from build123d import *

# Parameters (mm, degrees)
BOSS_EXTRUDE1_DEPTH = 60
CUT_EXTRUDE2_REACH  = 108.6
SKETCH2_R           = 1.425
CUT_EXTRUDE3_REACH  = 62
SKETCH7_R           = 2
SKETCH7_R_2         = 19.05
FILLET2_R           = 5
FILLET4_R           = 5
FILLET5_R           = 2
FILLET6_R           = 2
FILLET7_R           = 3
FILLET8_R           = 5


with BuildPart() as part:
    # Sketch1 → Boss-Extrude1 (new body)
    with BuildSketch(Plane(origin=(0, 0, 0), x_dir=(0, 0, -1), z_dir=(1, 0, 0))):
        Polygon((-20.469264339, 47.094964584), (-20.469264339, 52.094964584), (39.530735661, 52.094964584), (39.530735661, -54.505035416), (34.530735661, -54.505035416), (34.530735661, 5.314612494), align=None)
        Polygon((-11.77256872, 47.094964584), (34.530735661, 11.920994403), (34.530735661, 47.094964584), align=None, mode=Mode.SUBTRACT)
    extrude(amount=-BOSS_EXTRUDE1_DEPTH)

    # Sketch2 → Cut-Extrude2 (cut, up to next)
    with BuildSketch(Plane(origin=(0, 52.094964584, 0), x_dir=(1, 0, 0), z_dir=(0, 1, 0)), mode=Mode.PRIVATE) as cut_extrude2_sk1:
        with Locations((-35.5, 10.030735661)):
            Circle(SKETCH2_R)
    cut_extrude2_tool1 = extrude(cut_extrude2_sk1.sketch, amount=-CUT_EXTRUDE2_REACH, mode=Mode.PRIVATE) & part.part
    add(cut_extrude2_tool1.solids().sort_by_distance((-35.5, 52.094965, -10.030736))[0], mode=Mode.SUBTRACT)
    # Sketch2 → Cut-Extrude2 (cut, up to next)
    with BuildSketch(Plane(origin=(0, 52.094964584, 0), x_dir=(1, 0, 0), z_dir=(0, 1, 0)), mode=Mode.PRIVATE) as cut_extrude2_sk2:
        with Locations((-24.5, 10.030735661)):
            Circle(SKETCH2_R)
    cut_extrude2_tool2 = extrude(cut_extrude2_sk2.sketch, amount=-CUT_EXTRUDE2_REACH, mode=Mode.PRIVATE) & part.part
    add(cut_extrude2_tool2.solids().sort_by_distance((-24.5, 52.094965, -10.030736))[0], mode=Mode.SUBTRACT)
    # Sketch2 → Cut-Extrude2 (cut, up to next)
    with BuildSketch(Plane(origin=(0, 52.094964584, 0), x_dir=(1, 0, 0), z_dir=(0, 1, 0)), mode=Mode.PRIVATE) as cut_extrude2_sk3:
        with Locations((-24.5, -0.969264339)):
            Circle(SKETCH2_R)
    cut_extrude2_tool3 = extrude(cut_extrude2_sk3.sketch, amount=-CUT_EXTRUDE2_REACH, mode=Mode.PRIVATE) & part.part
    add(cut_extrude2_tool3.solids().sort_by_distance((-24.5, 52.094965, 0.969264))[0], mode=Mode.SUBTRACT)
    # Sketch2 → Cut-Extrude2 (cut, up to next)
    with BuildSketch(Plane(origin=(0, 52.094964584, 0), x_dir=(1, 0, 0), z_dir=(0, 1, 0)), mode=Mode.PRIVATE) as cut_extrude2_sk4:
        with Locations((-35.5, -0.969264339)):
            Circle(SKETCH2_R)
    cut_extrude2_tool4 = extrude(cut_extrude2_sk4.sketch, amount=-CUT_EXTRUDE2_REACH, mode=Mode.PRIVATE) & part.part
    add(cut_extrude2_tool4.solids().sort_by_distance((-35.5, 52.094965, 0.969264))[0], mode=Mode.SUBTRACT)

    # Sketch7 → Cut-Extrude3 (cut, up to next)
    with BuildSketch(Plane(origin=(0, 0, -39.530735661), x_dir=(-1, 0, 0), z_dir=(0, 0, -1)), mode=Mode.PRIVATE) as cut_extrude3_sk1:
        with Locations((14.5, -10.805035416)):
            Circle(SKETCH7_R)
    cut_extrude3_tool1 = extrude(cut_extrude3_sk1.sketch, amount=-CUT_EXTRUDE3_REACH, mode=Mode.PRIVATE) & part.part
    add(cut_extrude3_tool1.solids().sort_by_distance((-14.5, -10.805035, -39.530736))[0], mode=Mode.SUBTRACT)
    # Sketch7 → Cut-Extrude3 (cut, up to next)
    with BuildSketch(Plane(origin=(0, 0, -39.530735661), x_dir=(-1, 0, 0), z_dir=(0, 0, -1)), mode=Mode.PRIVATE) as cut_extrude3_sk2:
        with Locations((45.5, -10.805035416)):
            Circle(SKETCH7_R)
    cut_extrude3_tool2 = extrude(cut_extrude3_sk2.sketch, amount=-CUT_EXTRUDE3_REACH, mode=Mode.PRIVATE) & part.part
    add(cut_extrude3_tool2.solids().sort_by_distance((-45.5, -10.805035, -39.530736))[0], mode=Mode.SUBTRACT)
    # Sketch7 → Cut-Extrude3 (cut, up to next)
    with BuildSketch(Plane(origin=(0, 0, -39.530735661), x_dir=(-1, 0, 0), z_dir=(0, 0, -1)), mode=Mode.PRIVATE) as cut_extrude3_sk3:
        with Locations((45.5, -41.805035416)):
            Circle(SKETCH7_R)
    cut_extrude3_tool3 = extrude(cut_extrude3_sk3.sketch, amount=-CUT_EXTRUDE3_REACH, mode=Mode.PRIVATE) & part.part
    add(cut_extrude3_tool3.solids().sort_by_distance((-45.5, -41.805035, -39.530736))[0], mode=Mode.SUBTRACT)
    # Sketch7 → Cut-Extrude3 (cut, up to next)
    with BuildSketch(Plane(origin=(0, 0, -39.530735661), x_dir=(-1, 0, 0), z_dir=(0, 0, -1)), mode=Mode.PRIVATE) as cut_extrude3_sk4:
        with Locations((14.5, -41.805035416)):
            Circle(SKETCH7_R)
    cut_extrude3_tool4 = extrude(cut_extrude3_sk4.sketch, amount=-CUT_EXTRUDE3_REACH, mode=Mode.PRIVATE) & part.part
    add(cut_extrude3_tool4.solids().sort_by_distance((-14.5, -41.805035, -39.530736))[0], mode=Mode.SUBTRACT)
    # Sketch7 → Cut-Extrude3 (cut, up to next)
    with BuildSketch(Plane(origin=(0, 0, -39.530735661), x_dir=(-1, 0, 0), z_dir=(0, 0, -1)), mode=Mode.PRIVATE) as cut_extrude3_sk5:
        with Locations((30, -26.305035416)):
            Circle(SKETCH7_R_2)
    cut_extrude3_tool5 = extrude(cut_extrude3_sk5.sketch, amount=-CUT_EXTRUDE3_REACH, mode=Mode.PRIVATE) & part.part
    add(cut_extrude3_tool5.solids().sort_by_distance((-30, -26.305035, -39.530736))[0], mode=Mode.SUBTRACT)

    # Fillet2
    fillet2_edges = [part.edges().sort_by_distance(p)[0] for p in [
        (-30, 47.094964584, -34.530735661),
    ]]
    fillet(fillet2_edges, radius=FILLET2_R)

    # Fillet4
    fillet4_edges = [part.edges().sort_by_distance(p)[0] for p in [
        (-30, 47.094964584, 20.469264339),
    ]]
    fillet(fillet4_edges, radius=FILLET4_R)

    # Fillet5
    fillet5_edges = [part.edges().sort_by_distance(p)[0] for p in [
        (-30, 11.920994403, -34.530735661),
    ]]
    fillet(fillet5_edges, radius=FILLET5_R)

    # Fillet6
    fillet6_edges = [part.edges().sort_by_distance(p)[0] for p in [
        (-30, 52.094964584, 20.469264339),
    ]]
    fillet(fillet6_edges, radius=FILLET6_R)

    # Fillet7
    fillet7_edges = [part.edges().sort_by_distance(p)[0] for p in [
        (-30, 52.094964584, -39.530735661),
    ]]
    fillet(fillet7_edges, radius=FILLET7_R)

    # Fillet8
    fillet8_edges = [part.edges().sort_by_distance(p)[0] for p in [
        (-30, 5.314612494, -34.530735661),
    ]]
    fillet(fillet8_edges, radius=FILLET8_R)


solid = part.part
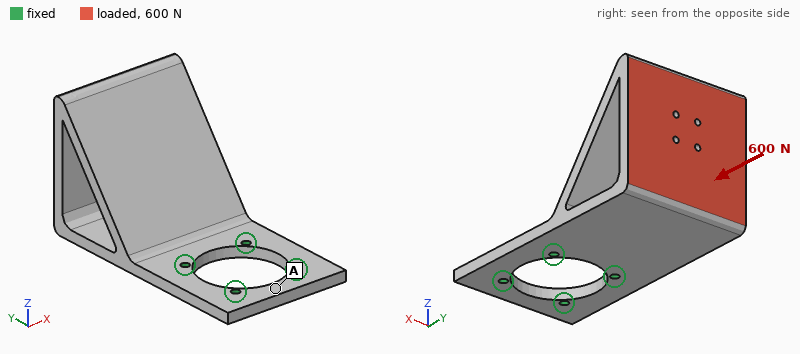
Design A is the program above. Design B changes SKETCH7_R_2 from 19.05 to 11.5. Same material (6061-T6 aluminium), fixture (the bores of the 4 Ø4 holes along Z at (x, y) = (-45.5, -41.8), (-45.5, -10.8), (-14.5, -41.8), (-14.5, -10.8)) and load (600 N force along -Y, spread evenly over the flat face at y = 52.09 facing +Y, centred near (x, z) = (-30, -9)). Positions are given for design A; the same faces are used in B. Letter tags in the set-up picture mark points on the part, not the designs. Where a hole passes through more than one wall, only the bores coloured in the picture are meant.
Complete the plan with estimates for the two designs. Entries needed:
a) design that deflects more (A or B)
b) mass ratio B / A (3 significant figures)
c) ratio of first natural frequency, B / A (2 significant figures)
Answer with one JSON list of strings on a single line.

["A", "1.06", "1.1"]
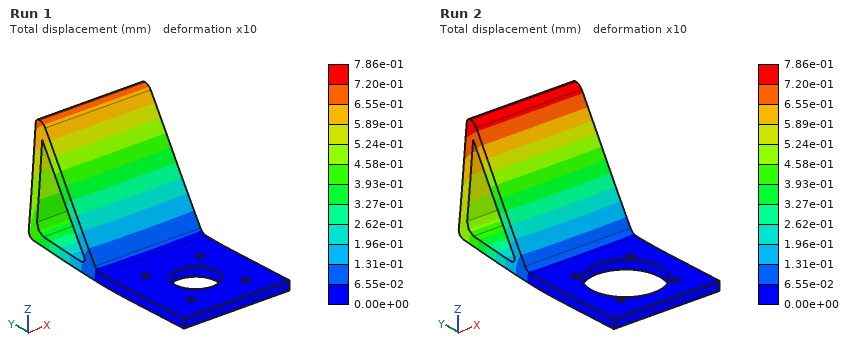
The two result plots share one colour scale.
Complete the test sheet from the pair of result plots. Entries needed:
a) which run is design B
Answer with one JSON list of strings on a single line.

["Run 1"]
